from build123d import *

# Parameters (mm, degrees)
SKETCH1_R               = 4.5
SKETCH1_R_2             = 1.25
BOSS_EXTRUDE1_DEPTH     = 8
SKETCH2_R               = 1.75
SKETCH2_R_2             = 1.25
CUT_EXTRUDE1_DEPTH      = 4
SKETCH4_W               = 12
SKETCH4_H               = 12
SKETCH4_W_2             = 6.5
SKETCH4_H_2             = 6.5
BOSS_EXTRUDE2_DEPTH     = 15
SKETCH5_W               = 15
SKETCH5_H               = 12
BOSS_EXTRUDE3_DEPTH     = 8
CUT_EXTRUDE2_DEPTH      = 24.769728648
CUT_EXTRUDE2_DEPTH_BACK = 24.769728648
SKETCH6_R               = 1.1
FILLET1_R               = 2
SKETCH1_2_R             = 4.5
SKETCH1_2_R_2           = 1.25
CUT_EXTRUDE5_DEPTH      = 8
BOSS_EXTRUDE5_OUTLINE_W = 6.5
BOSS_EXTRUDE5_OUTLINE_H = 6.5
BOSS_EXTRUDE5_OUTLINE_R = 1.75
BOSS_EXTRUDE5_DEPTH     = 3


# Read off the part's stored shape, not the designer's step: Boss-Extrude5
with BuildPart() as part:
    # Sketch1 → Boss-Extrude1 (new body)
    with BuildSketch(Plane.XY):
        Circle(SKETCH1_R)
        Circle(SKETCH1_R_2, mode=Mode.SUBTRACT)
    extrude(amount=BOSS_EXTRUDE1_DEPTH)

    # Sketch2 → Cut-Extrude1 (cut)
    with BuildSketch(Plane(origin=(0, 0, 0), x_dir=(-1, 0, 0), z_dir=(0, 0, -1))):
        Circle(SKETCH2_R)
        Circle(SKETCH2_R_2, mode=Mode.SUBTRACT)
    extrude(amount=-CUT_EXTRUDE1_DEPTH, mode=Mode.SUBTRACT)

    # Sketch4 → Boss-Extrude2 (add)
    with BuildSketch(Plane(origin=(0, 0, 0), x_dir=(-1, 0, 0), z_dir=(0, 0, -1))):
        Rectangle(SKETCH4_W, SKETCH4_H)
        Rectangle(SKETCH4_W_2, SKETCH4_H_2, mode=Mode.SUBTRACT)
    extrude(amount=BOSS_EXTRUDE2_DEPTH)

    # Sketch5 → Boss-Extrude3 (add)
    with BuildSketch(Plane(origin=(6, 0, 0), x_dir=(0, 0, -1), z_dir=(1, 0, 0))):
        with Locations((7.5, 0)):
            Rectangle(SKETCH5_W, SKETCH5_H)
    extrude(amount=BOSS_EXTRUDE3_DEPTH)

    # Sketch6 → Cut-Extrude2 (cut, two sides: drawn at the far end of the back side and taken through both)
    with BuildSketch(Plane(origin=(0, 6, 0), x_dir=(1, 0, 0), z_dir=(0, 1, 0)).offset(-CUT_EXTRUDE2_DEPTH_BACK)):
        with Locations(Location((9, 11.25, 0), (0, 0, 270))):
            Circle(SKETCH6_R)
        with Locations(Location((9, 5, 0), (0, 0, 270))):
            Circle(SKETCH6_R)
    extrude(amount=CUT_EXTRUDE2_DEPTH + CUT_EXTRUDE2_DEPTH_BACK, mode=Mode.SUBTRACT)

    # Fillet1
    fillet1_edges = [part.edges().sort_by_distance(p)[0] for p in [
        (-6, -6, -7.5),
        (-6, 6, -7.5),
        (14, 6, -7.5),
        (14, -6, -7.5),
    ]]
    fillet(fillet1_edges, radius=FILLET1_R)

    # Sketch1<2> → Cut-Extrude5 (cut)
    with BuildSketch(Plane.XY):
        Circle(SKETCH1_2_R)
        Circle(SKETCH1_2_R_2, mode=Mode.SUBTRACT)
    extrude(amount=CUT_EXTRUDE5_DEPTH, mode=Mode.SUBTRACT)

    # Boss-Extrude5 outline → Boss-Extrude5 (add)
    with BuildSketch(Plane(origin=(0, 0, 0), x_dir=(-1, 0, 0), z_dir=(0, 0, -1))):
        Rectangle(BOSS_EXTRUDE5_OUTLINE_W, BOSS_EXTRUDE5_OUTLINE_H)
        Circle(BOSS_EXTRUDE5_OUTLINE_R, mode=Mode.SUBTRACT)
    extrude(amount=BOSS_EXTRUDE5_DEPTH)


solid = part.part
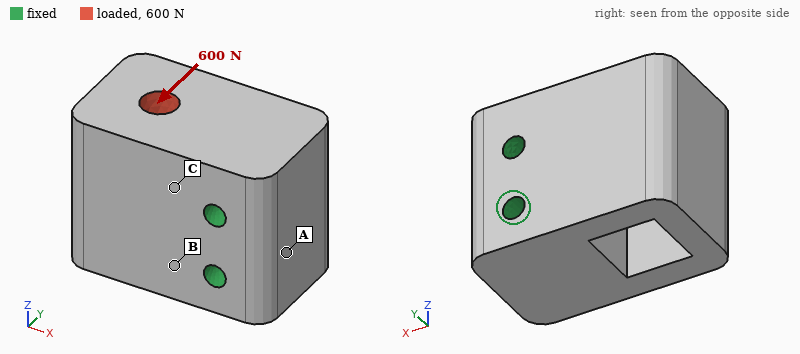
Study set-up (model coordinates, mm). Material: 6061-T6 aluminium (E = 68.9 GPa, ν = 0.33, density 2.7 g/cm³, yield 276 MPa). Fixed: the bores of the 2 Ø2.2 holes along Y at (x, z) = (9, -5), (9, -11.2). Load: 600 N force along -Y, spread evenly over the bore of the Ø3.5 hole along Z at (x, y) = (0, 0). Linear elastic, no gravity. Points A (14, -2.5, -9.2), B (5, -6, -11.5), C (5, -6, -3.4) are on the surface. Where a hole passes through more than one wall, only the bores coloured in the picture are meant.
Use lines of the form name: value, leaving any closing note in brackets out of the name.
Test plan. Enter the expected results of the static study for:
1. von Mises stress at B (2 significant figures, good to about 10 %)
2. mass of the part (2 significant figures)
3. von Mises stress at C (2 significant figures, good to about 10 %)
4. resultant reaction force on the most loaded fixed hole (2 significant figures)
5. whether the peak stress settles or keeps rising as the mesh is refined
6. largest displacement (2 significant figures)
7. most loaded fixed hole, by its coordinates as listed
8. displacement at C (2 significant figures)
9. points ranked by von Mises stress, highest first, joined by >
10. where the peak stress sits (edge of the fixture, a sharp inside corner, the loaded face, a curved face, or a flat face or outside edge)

von Mises stress at B: 14 MPa
mass of the part: 7.9 g
von Mises stress at C: 22 MPa
resultant reaction force on the most loaded fixed hole: 540 N
whether the peak stress settles or keeps rising as the mesh is refined: keeps rising
largest displacement: 8.5 µm
most loaded fixed hole, by its coordinates as listed: (9, -5)
displacement at C: 2.3 µm
points ranked by von Mises stress, highest first, joined by >: C > B > A
where the peak stress sits: edge of the fixture
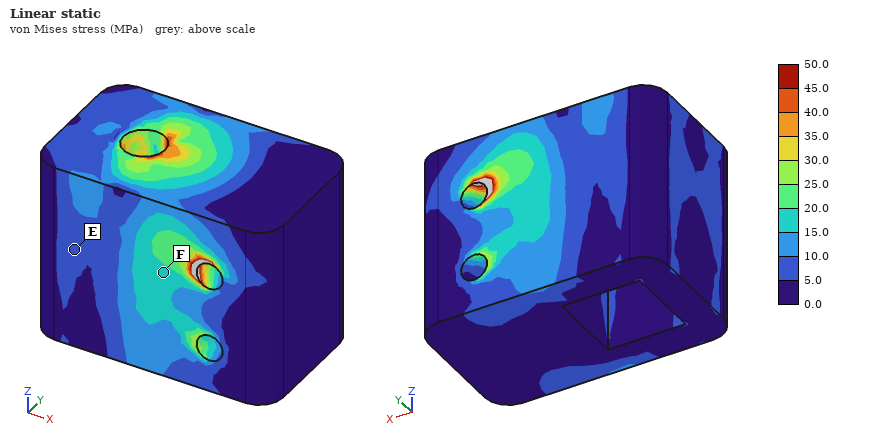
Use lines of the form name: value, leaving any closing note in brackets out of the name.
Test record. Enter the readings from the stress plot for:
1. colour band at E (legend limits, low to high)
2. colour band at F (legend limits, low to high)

colour band at E: 5.0 to 10.0 MPa
colour band at F: 15.0 to 20.0 MPa
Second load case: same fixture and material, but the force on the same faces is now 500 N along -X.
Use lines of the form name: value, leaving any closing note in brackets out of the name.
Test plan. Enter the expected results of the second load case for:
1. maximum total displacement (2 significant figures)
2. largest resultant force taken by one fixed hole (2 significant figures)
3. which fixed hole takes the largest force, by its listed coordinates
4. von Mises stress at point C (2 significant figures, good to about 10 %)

maximum total displacement: 3.7 µm
largest resultant force taken by one fixed hole: 670 N
which fixed hole takes the largest force, by its listed coordinates: (9, -5)
von Mises stress at point C: 8.7 MPa
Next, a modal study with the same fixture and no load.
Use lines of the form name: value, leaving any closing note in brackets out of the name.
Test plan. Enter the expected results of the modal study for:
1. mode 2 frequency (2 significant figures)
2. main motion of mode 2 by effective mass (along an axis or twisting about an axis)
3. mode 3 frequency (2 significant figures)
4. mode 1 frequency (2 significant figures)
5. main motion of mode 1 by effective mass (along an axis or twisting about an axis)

mode 2 frequency: 29 kHz
main motion of mode 2 by effective mass: along Z
mode 3 frequency: 43 kHz
mode 1 frequency: 24 kHz
main motion of mode 1 by effective mass: along Y
